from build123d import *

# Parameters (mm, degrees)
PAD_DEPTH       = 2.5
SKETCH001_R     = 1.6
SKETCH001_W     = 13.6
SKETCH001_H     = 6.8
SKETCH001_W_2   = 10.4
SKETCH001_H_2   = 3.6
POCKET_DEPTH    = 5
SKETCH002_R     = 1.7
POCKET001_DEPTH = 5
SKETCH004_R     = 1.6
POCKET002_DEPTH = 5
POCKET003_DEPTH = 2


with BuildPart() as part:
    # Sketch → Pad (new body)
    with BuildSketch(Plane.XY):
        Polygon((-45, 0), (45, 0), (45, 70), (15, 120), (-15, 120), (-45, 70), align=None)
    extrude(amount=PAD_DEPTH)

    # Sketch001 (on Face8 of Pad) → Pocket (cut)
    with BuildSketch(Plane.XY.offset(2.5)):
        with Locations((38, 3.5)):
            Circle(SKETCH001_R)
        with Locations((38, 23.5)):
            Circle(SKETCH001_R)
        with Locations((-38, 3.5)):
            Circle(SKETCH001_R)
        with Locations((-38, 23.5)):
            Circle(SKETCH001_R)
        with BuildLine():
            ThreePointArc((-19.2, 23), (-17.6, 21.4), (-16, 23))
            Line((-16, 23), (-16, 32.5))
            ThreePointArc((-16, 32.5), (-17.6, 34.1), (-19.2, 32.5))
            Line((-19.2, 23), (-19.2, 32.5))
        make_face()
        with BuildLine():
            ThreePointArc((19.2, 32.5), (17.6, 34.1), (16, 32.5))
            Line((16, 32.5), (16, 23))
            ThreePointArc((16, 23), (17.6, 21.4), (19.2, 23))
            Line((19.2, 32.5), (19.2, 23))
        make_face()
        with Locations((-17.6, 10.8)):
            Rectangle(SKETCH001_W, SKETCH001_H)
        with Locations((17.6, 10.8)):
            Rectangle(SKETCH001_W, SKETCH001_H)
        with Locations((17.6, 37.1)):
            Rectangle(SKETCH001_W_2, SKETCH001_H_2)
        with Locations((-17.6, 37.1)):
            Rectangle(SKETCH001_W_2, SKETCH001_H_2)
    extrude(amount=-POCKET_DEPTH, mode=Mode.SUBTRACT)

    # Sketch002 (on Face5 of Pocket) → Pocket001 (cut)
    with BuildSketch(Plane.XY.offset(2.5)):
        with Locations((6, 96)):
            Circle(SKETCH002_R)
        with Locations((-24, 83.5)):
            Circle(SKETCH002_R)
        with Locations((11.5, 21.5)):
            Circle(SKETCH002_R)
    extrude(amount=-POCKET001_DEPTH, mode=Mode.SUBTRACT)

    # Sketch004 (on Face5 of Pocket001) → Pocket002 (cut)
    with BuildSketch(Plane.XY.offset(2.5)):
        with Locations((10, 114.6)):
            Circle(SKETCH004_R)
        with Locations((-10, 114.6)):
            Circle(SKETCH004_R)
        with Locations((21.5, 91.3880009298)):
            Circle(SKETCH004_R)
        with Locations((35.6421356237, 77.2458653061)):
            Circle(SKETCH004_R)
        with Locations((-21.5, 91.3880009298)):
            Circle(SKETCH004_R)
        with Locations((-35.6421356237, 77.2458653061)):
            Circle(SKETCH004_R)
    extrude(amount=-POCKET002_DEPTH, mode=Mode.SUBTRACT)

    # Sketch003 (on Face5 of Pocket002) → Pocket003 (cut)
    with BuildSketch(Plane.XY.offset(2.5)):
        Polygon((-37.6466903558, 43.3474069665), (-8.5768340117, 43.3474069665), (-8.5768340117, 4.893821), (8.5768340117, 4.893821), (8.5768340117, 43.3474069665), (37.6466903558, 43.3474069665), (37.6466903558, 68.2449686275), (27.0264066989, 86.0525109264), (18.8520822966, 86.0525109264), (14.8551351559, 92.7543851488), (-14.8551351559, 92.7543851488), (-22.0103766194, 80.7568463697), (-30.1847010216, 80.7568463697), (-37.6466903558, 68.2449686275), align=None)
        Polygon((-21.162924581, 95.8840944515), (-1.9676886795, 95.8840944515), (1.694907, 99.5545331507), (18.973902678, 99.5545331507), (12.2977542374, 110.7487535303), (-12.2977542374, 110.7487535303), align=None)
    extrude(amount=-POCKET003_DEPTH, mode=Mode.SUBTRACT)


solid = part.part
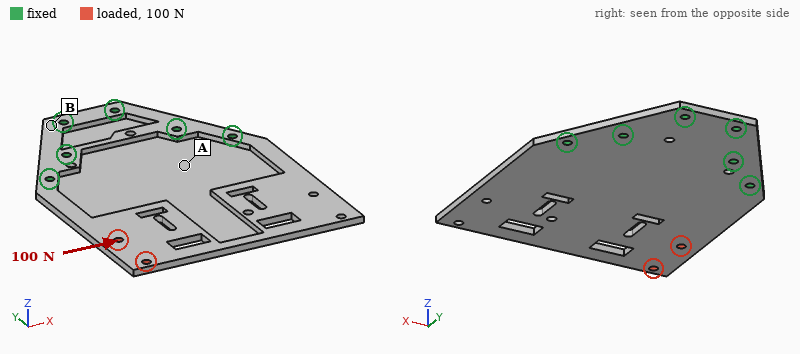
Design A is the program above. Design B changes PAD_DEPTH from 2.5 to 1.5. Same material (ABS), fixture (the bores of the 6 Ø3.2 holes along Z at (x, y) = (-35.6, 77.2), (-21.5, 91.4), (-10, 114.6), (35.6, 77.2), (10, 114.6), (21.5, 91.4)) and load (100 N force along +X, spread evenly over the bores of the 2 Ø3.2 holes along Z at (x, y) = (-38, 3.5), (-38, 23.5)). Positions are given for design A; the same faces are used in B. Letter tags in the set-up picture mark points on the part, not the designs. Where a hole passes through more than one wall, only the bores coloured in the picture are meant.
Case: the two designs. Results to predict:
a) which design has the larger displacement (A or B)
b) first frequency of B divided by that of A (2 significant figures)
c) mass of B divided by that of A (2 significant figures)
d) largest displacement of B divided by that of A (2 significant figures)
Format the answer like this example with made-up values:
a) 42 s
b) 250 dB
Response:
a) B
b) 0.62
c) 0.66
d) 1.7
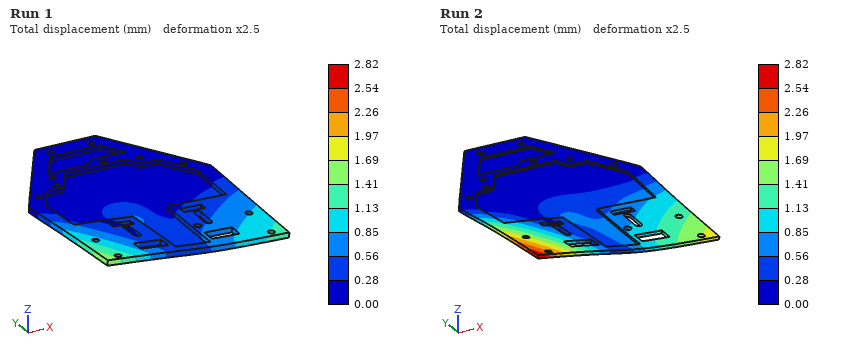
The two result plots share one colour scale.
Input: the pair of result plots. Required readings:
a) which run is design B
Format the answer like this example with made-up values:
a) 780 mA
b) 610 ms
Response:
a) Run 2
